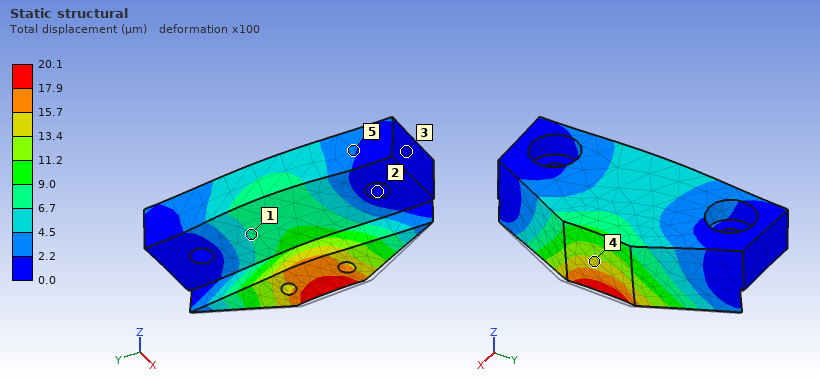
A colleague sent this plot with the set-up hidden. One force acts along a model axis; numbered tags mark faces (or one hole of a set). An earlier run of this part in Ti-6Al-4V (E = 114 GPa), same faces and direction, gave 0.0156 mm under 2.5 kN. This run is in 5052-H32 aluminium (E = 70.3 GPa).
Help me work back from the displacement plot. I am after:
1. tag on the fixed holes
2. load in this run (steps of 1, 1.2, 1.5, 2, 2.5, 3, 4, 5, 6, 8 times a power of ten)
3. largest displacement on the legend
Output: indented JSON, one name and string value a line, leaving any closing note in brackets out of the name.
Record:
{
  "tag on the fixed holes": "2",
  "load in this run": "2 kN",
  "largest displacement on the legend": "20.1 µm"
}
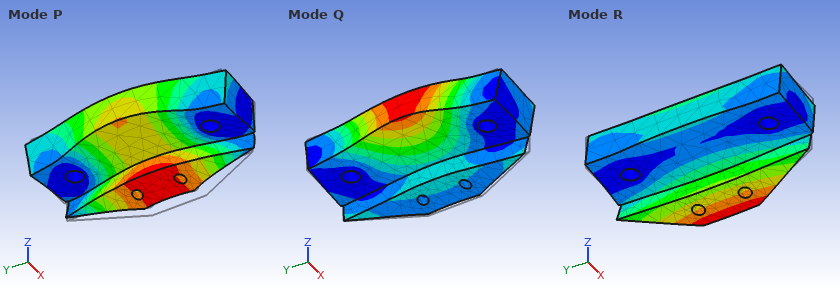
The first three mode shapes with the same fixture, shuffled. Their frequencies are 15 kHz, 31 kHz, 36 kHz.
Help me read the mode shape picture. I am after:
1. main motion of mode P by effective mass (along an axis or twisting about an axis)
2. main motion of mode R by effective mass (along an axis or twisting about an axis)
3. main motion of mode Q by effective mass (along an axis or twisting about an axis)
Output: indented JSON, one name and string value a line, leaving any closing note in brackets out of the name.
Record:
{
  "main motion of mode P by effective mass": "along X",
  "main motion of mode R by effective mass": "along Z",
  "main motion of mode Q by effective mass": "along Z"
}
